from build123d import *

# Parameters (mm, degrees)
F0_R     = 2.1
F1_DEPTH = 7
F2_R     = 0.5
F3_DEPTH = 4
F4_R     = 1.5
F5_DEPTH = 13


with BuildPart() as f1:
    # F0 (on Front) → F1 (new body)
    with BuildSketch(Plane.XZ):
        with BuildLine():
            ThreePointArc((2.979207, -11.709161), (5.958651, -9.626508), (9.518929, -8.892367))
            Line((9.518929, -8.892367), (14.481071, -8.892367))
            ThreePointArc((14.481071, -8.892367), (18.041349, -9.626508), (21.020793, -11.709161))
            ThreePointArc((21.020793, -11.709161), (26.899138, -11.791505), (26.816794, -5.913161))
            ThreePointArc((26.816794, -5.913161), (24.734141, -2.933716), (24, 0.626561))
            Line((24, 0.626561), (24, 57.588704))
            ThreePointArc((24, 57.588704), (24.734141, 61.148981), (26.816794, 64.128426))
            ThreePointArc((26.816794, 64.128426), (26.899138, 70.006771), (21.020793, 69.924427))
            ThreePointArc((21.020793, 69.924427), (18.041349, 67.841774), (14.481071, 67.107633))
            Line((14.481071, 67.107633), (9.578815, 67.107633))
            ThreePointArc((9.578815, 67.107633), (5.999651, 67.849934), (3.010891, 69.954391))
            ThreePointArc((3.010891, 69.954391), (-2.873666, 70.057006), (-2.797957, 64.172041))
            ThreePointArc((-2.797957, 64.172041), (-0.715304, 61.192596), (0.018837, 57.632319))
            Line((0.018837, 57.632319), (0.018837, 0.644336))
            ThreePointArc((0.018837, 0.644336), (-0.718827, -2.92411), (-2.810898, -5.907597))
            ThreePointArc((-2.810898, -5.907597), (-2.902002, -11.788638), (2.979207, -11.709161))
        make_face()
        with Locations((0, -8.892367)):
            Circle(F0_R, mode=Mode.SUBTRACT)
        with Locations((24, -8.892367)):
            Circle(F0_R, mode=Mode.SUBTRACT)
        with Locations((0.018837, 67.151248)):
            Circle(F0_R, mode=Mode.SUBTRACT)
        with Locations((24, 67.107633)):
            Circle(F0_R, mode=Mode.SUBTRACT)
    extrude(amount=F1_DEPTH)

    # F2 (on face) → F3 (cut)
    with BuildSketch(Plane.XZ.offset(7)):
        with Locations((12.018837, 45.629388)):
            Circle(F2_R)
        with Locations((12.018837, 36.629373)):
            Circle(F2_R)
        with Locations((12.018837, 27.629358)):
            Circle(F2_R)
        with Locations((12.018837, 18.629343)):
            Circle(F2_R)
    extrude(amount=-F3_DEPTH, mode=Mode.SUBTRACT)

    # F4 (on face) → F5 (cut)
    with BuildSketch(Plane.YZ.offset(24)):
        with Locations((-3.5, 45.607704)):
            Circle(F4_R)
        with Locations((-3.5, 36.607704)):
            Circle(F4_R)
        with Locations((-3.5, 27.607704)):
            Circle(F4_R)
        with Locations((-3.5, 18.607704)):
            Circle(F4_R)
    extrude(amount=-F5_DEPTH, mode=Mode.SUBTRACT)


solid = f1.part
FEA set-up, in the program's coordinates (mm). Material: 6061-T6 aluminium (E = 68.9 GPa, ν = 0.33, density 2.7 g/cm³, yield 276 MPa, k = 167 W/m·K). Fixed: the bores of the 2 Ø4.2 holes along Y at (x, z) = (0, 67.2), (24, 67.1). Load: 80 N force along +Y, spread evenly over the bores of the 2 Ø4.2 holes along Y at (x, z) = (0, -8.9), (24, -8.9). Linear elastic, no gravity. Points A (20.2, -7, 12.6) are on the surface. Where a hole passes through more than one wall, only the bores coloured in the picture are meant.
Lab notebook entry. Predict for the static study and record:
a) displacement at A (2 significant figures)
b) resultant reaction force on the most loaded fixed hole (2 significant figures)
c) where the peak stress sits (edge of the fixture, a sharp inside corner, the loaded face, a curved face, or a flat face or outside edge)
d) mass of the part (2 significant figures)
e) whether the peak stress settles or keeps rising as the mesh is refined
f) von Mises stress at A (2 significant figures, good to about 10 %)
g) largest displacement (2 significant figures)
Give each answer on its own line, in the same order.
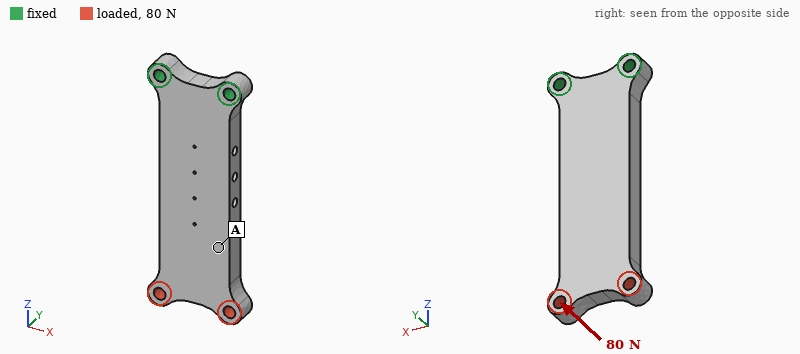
0.16 mm
40 N
edge of the fixture
36 g
keeps rising
8.7 MPa
0.29 mm
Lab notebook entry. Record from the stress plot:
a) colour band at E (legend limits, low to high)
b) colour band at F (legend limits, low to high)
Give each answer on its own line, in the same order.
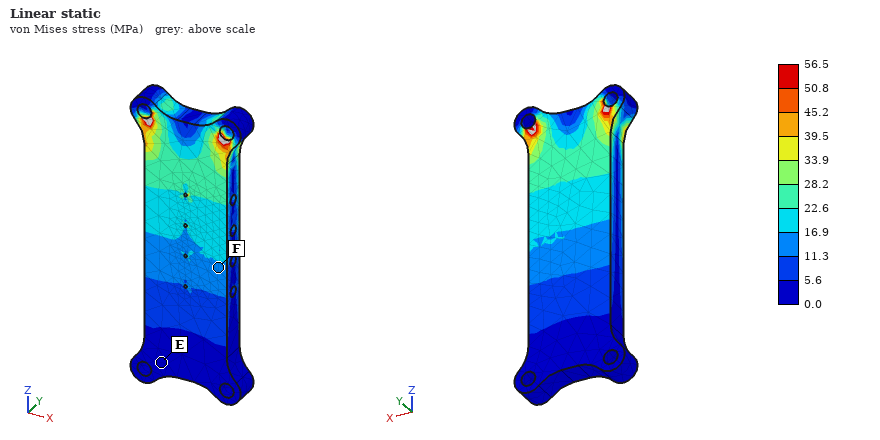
0.0 to 5.6 MPa
11.3 to 16.9 MPa
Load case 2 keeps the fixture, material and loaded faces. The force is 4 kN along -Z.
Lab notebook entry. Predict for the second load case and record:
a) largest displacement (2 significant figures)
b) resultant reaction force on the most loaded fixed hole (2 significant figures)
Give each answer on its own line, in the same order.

60 µm
2.2 kN
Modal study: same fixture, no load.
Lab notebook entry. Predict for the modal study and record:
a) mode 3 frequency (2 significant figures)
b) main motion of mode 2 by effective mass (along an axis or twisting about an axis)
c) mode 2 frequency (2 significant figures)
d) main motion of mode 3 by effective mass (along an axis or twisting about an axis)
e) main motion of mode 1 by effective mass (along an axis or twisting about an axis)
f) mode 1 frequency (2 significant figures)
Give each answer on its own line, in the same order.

5000 Hz
along X
3000 Hz
twisting about Z
along Y
880 Hz
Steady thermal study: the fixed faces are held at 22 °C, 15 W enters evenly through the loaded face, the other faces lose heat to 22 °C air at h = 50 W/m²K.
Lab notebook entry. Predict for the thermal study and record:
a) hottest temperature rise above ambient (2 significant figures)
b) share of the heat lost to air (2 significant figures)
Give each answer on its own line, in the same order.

38 K
33 %
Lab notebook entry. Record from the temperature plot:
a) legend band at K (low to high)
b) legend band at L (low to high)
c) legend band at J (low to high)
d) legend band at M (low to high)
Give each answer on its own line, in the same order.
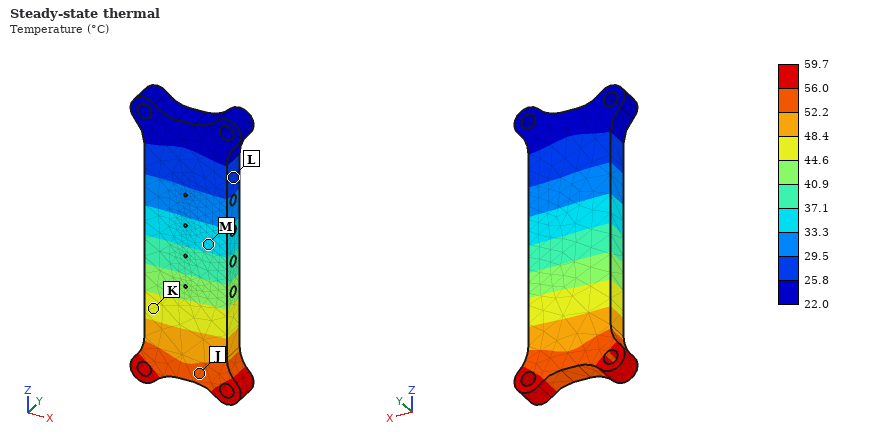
44.6 to 48.4 °C
25.8 to 29.5 °C
52.2 to 56.0 °C
33.3 to 37.1 °C
